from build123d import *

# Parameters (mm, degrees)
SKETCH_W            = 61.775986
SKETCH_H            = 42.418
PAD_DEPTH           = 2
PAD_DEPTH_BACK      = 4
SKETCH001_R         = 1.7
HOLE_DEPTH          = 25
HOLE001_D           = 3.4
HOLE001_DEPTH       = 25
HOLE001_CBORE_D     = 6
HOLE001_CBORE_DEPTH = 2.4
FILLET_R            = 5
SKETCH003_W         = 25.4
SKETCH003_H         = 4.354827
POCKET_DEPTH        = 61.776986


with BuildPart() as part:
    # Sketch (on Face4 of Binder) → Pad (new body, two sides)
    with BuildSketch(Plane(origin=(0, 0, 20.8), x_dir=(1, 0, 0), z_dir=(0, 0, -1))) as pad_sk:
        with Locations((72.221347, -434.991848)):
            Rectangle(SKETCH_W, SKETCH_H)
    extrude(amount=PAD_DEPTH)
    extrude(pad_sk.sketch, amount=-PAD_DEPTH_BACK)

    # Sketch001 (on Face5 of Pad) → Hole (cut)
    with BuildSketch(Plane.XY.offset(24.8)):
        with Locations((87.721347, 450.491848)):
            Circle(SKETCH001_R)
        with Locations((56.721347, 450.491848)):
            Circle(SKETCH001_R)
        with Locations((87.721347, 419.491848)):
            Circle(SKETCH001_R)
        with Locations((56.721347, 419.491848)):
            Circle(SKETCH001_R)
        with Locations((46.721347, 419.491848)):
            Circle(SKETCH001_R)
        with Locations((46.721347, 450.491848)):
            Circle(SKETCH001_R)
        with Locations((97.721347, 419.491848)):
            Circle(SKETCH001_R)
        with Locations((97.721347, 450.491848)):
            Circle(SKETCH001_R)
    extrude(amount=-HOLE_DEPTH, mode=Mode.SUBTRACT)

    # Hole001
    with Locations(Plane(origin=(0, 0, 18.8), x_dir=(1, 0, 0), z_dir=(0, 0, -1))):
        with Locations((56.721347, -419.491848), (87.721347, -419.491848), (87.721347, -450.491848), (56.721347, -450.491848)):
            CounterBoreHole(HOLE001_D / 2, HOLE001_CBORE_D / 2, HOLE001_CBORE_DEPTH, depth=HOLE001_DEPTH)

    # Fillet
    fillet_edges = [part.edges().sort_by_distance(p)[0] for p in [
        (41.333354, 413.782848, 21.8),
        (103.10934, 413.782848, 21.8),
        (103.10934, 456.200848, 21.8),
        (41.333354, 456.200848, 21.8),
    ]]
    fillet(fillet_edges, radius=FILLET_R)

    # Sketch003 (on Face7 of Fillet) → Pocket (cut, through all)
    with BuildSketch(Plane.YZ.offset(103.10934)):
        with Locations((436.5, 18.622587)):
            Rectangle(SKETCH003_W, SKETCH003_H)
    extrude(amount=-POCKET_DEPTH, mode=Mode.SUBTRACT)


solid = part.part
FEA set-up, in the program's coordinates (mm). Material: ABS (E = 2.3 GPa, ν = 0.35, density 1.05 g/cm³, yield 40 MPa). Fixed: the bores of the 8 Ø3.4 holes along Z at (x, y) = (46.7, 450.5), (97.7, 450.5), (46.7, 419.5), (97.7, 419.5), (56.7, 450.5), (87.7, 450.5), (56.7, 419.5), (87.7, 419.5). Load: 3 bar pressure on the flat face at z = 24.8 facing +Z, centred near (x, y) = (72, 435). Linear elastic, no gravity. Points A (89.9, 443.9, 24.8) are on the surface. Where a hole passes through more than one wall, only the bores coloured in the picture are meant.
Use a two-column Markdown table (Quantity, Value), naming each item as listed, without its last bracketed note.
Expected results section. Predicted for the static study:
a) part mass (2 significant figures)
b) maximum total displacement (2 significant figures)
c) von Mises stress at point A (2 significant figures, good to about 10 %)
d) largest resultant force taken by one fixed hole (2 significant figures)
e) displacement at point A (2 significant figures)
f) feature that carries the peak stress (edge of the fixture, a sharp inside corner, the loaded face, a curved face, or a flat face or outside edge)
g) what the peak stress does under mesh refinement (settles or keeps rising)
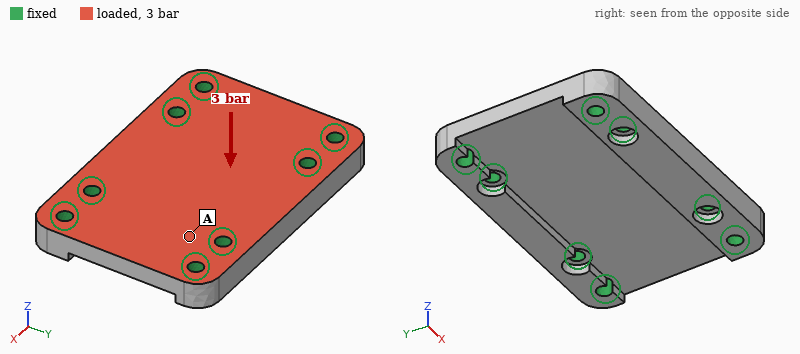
| Quantity | Value |
|---|---|
| part mass | 12 g |
| maximum total displacement | 0.12 mm |
| von Mises stress at point A | 2.1 MPa |
| largest resultant force taken by one fixed hole | 140 N |
| displacement at point A | 0.036 mm |
| feature that carries the peak stress | edge of the fixture |
| what the peak stress does under mesh refinement | keeps rising |
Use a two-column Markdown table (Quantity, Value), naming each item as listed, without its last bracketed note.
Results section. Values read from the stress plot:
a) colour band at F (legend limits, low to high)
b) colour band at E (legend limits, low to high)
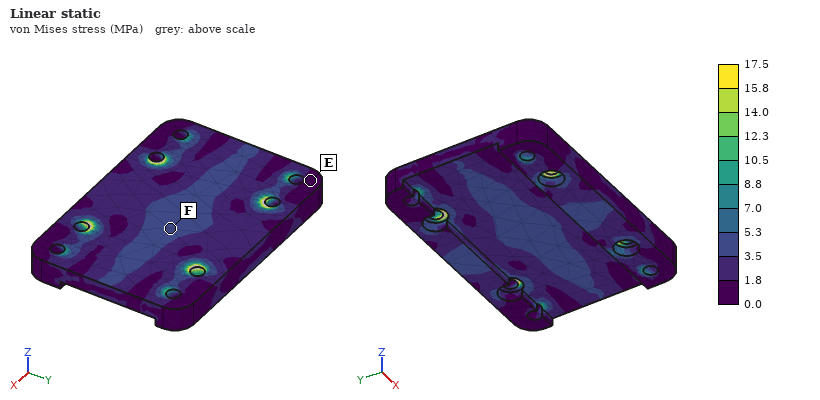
| Quantity | Value |
|---|---|
| colour band at F | 3.5 to 5.3 MPa |
| colour band at E | 0.0 to 1.8 MPa |
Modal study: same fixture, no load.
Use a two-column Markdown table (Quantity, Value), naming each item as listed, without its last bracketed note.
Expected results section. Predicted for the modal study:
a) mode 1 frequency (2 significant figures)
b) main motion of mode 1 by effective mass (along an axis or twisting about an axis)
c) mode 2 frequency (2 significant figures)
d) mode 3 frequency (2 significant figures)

| Quantity | Value |
|---|---|
| mode 1 frequency | 4600 Hz |
| main motion of mode 1 by effective mass | along Z |
| mode 2 frequency | 6800 Hz |
| mode 3 frequency | 6900 Hz |
